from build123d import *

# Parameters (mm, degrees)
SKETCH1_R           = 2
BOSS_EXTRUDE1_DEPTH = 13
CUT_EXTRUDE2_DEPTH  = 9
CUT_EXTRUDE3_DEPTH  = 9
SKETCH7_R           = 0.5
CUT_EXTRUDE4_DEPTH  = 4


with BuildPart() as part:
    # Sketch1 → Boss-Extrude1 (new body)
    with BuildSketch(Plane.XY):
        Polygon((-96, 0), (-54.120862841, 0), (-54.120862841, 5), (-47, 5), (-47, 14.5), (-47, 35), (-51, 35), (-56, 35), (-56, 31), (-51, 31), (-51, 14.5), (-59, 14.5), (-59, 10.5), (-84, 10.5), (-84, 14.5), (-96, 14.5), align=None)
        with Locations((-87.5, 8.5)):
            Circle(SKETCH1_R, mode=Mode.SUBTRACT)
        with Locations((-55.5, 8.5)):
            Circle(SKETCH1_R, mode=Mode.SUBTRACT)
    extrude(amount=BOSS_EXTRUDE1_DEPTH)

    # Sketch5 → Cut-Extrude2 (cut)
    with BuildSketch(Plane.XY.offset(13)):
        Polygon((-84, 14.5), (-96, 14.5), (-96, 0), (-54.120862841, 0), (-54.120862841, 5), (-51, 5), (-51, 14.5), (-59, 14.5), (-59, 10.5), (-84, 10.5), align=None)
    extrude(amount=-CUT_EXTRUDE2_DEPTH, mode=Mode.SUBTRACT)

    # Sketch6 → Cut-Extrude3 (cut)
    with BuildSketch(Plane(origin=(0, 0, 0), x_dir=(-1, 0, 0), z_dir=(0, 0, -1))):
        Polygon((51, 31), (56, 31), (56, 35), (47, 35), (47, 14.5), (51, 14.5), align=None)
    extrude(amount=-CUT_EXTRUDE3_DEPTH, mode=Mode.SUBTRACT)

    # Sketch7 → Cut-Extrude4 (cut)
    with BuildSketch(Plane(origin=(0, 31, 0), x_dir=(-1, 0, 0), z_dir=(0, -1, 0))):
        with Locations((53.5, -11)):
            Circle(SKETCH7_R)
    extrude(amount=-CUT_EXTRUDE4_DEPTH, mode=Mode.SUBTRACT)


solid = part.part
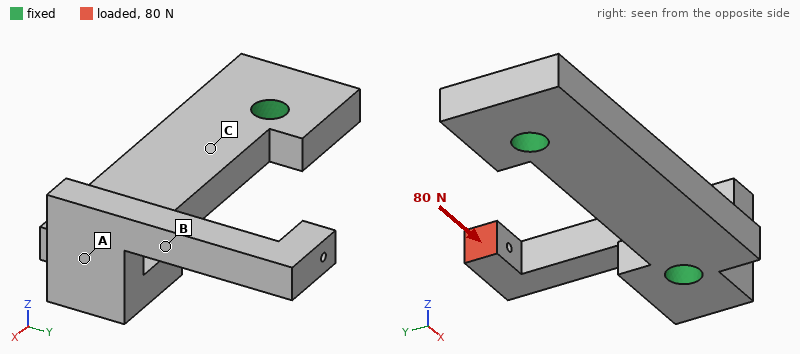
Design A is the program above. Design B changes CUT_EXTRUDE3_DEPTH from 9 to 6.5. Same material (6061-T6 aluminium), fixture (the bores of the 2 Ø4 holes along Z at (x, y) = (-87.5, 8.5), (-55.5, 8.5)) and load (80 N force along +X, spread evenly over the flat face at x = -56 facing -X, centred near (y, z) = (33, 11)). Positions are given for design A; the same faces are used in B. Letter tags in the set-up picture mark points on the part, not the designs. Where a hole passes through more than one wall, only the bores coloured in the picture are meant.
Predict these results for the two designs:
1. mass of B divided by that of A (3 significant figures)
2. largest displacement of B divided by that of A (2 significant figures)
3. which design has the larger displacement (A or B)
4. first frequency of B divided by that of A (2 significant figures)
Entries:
1.09
0.69
A
0.94
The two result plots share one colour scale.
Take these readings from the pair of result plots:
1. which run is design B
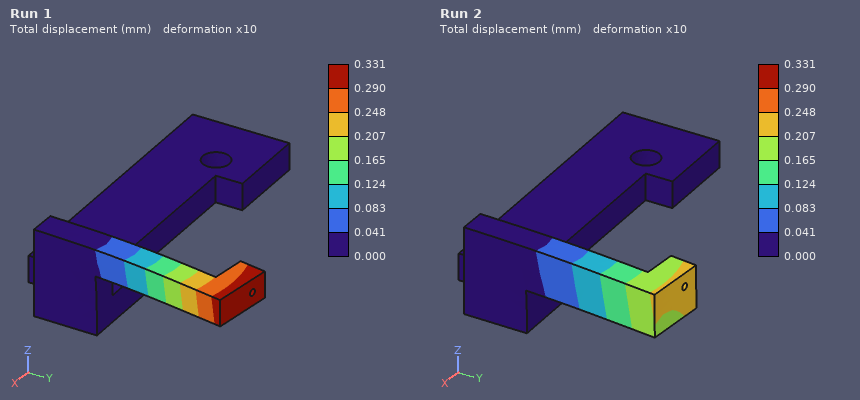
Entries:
Run 2
